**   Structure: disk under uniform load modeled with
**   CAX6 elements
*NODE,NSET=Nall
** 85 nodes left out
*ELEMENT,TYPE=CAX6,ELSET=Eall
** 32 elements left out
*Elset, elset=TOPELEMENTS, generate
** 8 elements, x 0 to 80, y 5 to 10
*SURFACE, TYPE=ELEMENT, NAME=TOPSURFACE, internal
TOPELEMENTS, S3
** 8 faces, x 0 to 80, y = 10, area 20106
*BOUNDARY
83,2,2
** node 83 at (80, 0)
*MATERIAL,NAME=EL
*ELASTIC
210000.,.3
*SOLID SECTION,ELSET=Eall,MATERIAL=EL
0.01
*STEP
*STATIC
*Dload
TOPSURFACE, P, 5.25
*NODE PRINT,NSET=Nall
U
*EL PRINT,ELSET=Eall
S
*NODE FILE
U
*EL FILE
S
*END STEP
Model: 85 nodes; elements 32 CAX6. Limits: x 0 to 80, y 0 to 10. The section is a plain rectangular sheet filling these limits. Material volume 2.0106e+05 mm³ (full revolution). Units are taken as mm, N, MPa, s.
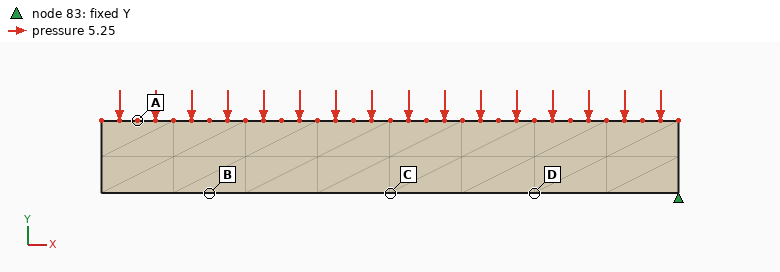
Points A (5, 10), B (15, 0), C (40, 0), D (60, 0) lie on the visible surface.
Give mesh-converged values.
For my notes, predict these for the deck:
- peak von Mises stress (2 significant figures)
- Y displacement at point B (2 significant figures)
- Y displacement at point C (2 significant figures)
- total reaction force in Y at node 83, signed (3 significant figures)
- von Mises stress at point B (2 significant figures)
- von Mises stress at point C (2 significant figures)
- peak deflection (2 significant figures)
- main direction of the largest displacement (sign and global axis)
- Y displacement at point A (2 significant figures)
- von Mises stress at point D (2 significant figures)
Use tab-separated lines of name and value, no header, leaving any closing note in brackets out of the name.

peak von Mises stress	420 MPa
Y displacement at point B	-0.69 mm
Y displacement at point C	-0.51 mm
total reaction force in Y at node 83, signed	1.06e+05 N
von Mises stress at point B	410 MPa
von Mises stress at point C	340 MPa
peak deflection	0.73 mm
main direction of the largest displacement	-Y
Y displacement at point A	-0.72 mm
von Mises stress at point D	250 MPa
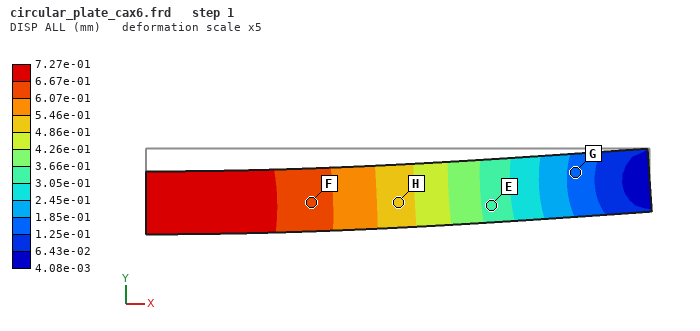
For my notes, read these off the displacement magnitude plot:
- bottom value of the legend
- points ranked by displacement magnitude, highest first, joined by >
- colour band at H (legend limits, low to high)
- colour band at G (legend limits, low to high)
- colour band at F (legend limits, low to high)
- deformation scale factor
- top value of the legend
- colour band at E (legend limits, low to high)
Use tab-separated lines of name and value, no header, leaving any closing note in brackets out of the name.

bottom value of the legend	4.08e-03 mm
points ranked by displacement magnitude, highest first, joined by >	F > H > E > G
colour band at H	4.86e-01 to 5.46e-01 mm
colour band at G	1.25e-01 to 1.85e-01 mm
colour band at F	6.07e-01 to 6.67e-01 mm
deformation scale factor	5
top value of the legend	7.27e-01 mm
colour band at E	3.05e-01 to 3.66e-01 mm
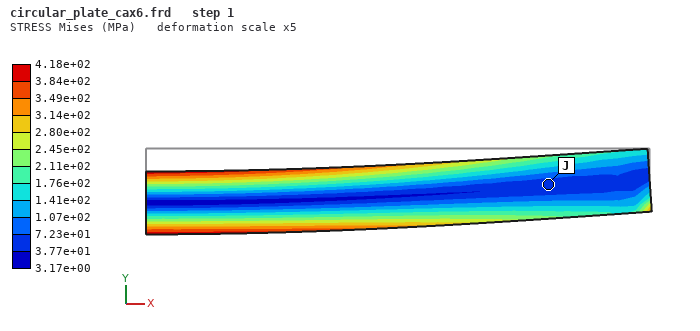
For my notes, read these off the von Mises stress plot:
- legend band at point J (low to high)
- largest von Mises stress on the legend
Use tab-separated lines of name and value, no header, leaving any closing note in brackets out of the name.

legend band at point J	3.77e+01 to 7.23e+01 MPa
largest von Mises stress on the legend	4.18e+02 MPa
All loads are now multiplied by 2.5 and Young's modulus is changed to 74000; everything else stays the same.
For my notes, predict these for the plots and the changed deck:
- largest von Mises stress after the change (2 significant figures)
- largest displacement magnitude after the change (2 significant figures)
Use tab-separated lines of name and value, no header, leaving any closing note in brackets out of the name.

largest von Mises stress after the change	1000 MPa
largest displacement magnitude after the change	5.2 mm
